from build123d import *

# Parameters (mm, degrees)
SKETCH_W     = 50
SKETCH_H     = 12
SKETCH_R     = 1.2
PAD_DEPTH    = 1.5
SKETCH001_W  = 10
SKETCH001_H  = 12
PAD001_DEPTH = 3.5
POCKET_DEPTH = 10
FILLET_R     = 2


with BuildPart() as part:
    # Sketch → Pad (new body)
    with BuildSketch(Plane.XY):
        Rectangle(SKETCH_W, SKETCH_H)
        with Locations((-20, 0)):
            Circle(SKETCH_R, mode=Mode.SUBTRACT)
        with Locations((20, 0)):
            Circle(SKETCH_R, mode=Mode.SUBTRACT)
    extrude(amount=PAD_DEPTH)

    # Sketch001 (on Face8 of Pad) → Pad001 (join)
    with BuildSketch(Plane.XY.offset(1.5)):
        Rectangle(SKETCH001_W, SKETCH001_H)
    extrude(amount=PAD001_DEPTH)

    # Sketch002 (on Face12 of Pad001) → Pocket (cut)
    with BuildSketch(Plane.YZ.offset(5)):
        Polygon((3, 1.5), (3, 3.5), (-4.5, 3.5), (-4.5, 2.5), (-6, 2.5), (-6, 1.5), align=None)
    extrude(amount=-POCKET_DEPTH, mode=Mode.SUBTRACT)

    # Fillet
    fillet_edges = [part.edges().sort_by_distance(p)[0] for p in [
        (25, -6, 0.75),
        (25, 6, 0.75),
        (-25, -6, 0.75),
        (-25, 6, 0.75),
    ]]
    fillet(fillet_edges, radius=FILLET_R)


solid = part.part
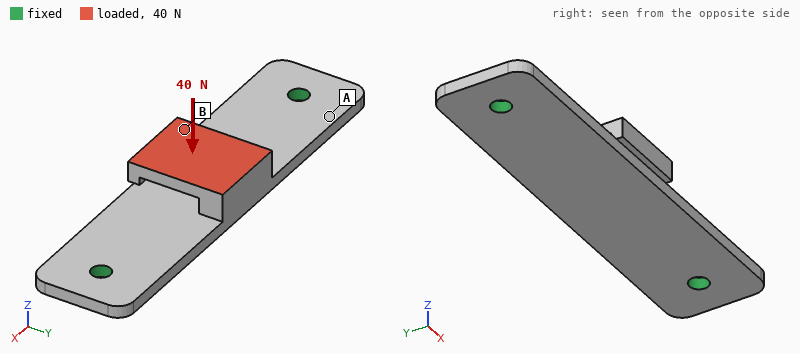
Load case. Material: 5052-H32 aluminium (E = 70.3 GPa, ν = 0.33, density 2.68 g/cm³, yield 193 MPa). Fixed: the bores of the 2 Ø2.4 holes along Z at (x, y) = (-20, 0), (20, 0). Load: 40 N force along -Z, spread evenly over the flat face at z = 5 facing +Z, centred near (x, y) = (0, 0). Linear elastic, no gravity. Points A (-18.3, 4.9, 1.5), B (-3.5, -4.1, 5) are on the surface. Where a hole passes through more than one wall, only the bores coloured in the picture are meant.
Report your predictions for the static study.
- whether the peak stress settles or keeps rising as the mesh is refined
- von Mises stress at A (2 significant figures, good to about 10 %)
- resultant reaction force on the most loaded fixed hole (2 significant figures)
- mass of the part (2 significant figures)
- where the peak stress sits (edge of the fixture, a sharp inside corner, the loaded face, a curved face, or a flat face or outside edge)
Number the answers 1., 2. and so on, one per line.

1. keeps rising
2. 19 MPa
3. 21 N
4. 3.0 g
5. edge of the fixture
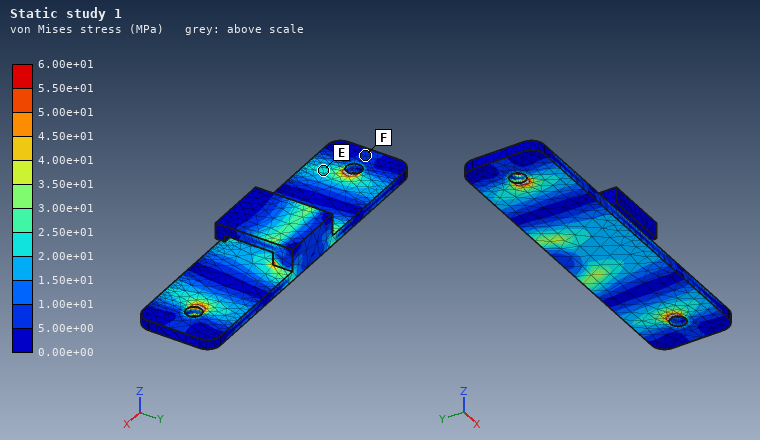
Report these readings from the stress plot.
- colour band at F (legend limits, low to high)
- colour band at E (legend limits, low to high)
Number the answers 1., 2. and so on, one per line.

1. 5.00e+00 to 1.00e+01 MPa
2. 2.00e+01 to 2.50e+01 MPa
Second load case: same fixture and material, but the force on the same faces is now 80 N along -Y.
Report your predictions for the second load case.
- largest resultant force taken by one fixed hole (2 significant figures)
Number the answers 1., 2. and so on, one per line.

1. 40 N
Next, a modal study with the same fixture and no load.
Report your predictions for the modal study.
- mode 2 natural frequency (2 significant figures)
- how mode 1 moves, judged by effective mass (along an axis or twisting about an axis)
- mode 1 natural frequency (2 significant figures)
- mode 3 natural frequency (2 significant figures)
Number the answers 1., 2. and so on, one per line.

1. 6000 Hz
2. along Z
3. 4200 Hz
4. 11 kHz
